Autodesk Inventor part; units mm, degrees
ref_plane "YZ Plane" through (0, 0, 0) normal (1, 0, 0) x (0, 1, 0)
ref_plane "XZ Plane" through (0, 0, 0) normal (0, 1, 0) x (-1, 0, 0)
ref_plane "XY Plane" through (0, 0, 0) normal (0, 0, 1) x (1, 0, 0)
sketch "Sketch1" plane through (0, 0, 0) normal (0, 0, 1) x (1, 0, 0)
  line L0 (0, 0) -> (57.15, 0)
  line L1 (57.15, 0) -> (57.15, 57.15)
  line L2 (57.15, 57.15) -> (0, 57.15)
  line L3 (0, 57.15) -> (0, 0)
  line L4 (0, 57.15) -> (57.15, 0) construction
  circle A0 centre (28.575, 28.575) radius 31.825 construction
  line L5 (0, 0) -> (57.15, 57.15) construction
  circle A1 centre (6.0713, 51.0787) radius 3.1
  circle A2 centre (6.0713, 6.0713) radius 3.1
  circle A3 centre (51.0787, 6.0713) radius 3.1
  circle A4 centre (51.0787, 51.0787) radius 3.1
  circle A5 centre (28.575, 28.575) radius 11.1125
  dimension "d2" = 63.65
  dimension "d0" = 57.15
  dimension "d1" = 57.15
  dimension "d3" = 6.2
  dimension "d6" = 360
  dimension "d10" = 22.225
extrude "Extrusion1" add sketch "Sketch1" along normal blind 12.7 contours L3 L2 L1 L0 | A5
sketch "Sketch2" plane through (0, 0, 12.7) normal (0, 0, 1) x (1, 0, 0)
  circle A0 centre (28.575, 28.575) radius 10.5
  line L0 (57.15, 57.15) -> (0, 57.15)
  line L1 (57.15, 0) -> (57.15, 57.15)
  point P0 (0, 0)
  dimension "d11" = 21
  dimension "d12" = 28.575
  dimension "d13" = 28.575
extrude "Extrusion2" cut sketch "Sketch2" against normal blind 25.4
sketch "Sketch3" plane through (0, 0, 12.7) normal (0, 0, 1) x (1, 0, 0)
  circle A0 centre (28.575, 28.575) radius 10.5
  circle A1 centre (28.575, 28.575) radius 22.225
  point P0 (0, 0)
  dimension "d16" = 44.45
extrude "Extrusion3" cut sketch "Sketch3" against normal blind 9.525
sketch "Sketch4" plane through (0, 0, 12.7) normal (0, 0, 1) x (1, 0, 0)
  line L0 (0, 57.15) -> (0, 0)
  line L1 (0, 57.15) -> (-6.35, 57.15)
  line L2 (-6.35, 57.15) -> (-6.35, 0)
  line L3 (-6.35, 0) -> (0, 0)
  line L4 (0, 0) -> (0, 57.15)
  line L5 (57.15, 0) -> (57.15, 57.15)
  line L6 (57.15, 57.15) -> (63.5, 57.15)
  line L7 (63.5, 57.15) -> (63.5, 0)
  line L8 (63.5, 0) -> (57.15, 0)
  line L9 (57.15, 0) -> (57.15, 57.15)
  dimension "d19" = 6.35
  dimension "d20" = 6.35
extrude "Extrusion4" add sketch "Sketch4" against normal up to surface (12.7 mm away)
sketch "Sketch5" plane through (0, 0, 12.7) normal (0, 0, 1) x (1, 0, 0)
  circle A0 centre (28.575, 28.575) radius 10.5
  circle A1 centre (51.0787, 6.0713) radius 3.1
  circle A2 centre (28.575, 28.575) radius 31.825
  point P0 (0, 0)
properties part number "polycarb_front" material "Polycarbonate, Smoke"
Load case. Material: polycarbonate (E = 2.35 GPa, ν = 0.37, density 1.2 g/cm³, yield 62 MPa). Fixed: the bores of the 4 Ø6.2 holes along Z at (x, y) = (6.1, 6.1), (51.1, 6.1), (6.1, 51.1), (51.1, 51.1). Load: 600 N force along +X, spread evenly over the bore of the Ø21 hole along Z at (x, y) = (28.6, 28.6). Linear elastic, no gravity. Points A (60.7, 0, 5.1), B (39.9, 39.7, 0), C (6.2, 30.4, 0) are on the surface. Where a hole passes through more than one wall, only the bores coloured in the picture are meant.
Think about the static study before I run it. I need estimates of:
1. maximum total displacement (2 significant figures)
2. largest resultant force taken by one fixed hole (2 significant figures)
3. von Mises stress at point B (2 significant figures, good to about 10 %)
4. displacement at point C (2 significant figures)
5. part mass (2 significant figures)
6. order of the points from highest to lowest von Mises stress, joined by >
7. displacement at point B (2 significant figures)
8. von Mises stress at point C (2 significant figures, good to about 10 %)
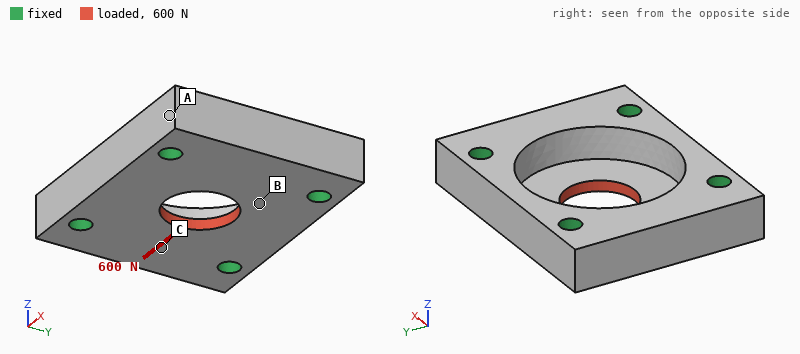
33 µm
150 N
2.3 MPa
20 µm
40 g
B > C > A
18 µm
1.3 MPa
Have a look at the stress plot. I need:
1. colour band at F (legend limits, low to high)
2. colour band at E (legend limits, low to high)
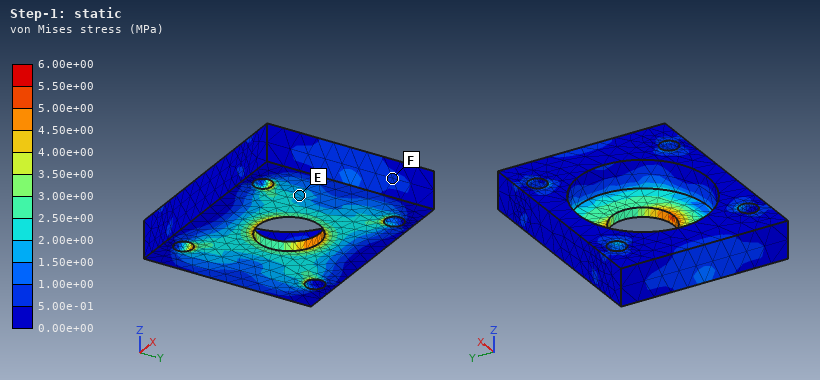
5.00e-01 to 1.00e+00 MPa
1.50e+00 to 2.00e+00 MPa
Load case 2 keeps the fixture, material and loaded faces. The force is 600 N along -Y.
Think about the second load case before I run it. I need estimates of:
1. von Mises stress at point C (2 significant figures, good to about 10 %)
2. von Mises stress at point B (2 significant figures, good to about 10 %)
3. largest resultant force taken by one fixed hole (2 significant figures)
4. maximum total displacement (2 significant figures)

0.85 MPa
2.5 MPa
160 N
40 µm
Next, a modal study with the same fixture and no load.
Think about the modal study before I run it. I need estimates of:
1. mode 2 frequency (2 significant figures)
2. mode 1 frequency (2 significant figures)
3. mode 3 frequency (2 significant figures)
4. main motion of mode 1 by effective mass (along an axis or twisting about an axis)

6000 Hz
4800 Hz
6000 Hz
along Z
